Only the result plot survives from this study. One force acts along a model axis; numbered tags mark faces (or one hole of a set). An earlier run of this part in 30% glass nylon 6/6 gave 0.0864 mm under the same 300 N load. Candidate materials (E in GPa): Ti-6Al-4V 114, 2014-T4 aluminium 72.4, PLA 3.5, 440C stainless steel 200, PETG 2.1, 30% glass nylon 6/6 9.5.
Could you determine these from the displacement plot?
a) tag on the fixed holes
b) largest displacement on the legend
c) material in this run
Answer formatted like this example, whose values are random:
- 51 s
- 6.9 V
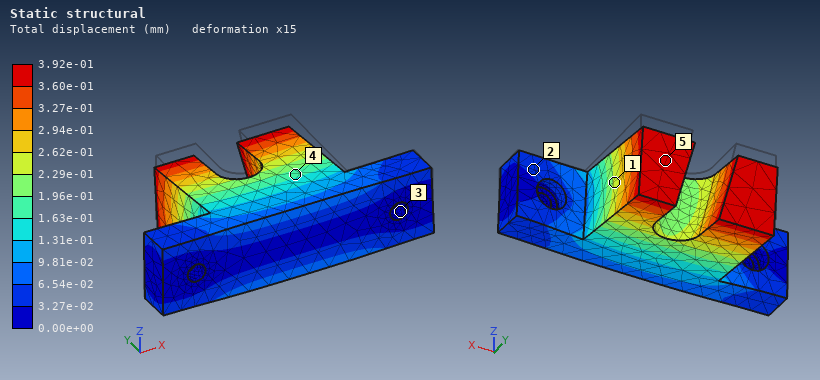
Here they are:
- 3
- 3.92e-01 mm
- PETG
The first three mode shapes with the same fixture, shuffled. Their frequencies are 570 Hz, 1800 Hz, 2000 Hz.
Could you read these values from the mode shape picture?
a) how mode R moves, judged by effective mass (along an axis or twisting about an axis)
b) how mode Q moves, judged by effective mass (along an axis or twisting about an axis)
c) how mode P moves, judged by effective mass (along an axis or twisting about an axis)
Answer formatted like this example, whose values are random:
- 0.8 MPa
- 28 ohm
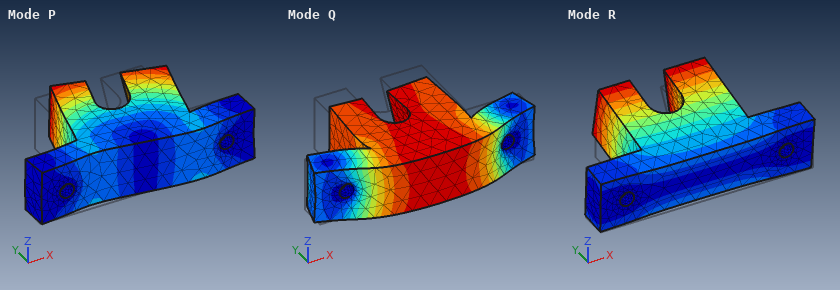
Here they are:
- along Z
- along Y
- along X
